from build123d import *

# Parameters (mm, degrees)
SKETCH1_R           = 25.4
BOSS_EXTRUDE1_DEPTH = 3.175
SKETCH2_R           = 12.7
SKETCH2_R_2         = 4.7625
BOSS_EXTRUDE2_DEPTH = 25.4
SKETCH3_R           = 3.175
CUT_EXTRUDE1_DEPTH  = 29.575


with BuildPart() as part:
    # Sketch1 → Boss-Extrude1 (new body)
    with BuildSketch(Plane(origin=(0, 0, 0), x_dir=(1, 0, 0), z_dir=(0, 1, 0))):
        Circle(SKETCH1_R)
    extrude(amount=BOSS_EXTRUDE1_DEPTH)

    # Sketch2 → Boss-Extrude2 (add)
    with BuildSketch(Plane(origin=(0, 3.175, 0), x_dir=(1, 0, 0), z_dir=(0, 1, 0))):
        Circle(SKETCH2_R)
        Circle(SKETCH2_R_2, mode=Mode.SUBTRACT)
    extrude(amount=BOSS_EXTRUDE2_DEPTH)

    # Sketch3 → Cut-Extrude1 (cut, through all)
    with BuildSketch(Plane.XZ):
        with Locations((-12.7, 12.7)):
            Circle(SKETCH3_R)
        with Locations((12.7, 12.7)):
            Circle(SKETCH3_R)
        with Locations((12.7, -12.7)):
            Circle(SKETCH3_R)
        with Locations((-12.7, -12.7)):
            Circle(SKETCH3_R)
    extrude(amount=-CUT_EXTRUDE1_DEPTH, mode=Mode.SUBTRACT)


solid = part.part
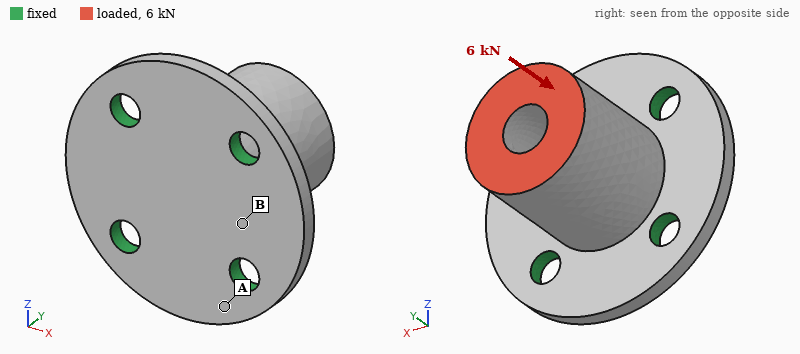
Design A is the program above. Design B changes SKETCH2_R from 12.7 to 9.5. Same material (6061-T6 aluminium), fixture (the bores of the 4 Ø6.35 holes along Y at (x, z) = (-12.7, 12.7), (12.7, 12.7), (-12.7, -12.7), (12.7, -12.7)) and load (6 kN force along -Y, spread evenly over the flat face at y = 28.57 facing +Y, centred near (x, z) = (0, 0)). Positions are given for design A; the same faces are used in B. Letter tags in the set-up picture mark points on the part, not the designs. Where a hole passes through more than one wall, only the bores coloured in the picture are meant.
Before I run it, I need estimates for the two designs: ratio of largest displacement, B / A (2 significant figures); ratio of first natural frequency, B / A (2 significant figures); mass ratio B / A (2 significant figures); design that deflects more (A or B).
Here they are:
2.5
0.82
0.67
B
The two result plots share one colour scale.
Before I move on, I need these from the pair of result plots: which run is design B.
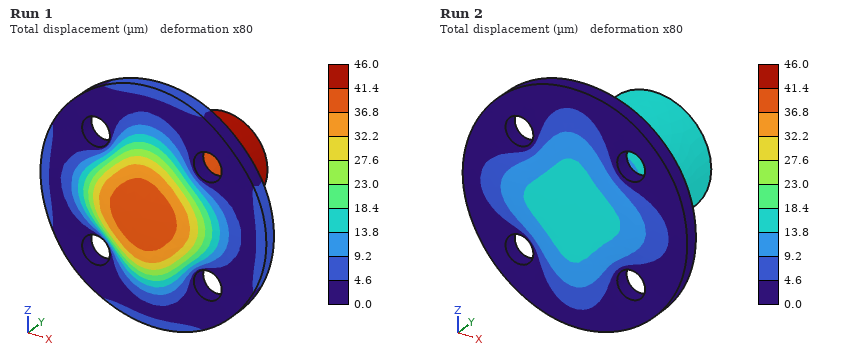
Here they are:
Run 1
